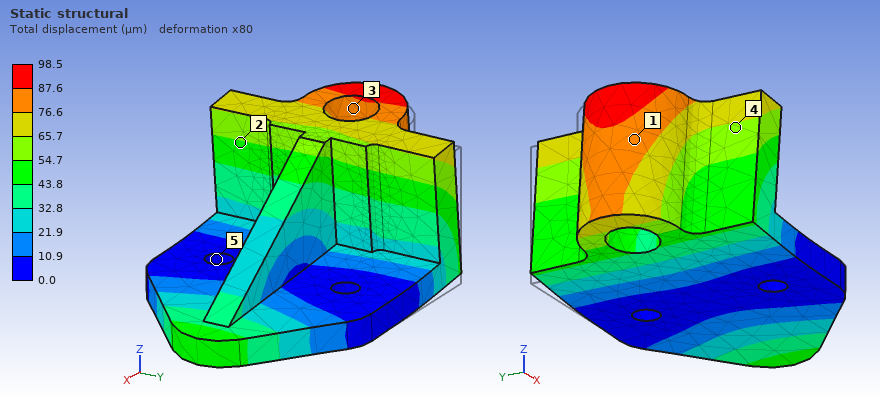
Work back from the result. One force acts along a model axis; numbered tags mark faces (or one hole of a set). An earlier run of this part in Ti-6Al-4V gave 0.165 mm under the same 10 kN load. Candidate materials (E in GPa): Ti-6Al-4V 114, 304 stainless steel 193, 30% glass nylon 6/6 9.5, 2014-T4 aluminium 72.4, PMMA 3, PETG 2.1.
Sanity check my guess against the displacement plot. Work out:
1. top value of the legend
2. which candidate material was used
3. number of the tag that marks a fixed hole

98.5 µm
304 stainless steel
5
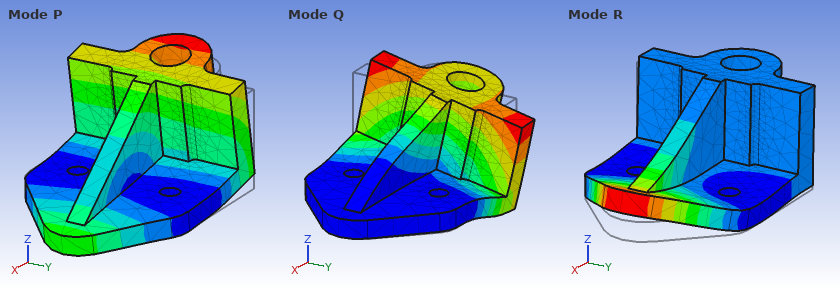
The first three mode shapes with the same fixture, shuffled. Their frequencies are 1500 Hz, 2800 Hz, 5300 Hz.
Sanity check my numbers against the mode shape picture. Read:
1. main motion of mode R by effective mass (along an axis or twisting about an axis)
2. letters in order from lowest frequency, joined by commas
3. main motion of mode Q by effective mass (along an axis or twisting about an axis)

along Z
P, Q, R
along Y
